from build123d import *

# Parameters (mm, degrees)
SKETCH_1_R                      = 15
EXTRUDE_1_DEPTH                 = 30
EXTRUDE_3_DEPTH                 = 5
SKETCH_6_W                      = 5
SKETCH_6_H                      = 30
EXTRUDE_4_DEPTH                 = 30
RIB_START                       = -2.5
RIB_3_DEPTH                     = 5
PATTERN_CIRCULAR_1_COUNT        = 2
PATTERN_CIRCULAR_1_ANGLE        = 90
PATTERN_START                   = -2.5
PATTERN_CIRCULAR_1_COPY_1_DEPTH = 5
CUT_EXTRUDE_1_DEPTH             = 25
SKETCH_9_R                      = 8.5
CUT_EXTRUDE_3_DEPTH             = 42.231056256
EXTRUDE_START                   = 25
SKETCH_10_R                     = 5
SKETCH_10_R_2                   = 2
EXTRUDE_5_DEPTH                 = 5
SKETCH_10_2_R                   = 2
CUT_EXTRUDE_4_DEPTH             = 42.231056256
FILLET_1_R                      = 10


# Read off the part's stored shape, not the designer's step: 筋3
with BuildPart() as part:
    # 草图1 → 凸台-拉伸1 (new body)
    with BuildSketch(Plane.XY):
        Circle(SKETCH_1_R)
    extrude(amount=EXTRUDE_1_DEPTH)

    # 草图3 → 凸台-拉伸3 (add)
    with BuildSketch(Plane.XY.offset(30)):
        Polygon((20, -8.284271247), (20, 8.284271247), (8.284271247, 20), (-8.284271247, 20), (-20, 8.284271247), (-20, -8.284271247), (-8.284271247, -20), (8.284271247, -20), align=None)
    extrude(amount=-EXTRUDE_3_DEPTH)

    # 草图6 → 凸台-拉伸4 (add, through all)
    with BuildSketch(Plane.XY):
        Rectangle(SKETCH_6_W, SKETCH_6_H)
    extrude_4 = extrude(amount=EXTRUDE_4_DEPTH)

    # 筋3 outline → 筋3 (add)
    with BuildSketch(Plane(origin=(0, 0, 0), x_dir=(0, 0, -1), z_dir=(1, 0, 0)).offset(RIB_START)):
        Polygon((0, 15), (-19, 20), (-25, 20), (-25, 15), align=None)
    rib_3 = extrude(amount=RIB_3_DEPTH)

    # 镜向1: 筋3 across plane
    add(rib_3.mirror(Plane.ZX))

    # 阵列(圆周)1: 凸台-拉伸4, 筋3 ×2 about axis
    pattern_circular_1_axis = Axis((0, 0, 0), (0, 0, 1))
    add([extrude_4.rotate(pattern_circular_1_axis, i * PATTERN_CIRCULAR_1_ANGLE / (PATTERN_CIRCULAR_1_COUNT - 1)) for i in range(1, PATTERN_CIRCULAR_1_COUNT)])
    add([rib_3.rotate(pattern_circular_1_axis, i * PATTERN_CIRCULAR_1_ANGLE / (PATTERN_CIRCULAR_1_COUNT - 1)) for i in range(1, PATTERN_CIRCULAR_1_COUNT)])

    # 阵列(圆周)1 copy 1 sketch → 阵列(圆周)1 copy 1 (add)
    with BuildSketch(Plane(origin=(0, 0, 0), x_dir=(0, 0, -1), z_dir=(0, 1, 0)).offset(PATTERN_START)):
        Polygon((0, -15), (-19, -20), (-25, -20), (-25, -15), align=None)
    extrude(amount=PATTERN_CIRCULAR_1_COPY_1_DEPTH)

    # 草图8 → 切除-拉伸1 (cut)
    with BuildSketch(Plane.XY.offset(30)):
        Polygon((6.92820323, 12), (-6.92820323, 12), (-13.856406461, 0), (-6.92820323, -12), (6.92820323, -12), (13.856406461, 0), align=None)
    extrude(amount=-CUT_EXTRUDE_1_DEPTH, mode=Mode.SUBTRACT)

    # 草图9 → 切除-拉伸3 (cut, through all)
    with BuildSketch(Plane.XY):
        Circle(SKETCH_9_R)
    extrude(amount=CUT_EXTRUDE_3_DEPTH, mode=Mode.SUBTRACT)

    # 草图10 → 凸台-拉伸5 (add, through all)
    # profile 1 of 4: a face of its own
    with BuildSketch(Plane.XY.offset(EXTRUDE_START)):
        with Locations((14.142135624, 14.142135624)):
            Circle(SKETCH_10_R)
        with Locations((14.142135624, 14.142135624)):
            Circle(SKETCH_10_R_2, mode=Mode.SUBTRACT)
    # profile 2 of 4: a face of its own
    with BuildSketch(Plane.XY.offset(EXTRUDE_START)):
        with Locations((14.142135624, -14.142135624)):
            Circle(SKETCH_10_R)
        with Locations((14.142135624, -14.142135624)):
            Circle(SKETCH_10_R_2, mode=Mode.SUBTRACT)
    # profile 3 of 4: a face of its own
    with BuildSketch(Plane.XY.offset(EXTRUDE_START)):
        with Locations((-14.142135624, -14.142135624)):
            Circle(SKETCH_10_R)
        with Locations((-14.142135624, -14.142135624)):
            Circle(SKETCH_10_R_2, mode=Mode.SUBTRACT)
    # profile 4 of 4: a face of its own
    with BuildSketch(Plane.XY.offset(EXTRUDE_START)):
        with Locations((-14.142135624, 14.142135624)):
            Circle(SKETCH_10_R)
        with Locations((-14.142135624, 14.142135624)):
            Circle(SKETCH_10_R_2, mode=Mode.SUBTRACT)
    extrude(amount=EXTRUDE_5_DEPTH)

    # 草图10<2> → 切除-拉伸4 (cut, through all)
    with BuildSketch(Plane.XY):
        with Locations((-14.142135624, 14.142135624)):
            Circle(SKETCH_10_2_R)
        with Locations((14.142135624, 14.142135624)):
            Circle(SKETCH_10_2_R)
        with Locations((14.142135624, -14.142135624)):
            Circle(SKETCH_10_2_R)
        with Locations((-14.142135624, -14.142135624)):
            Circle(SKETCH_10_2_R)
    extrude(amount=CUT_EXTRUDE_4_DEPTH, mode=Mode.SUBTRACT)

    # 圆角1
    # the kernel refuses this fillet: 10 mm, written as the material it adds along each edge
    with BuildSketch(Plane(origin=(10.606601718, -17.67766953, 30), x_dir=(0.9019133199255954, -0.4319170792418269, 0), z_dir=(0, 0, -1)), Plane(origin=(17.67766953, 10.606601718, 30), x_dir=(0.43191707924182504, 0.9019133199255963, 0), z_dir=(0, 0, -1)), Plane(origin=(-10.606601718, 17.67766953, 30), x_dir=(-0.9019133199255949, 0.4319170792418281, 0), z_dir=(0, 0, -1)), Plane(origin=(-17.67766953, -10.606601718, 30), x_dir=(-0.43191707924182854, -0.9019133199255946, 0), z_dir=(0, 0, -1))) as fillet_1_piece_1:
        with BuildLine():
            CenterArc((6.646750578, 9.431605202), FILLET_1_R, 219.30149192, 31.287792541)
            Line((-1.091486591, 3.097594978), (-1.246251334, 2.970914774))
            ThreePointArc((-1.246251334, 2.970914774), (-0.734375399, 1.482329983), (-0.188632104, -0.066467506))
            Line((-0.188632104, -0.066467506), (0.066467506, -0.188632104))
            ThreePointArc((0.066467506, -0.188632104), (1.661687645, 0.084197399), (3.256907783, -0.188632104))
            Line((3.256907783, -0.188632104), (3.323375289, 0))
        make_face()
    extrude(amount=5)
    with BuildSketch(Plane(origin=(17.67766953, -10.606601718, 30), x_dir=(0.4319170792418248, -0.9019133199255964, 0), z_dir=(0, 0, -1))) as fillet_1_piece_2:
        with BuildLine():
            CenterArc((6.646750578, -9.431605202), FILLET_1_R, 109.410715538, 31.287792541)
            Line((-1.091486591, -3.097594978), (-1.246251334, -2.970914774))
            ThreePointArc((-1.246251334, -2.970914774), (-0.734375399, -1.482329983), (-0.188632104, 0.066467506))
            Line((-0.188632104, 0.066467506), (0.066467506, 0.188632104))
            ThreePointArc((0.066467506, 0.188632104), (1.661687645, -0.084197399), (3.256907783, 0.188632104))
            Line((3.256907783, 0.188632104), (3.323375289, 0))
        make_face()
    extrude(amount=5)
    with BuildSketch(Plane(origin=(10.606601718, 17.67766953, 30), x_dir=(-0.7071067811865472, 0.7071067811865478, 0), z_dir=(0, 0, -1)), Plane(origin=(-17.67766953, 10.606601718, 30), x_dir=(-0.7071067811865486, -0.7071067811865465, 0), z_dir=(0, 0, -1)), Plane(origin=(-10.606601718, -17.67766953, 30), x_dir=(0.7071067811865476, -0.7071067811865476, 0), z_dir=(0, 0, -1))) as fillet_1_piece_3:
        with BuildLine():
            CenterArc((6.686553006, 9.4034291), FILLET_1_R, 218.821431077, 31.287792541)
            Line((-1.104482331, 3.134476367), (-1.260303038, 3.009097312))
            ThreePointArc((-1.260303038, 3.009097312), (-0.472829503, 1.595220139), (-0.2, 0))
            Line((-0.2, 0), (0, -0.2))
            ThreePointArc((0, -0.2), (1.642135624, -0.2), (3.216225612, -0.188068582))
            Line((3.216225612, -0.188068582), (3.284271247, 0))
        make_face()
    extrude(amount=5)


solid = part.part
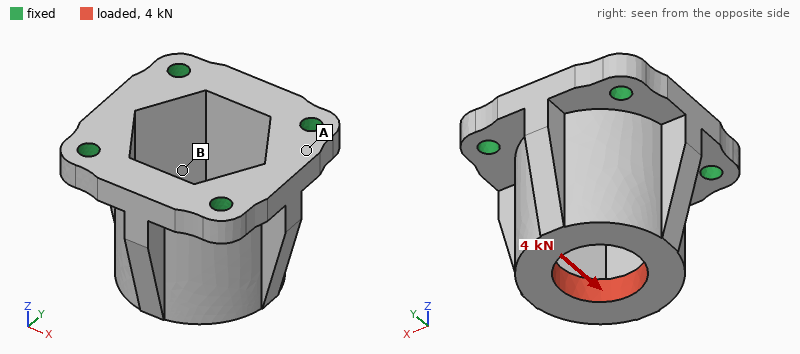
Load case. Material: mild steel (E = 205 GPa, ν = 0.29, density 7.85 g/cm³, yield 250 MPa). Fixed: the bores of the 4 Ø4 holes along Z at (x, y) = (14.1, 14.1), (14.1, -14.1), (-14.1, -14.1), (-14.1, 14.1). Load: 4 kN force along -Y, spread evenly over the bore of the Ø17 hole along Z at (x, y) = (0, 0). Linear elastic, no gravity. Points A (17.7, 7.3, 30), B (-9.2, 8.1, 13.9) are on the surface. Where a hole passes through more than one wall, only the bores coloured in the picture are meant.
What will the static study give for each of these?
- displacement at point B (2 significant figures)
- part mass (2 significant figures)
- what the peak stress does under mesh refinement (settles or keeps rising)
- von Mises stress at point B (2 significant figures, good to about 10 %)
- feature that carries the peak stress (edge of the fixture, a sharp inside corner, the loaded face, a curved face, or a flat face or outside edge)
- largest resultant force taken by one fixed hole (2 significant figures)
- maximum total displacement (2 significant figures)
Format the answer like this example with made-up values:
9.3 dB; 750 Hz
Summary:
12 µm; 100 g; keeps rising; 44 MPa; edge of the fixture; 2.2 kN; 27 µm
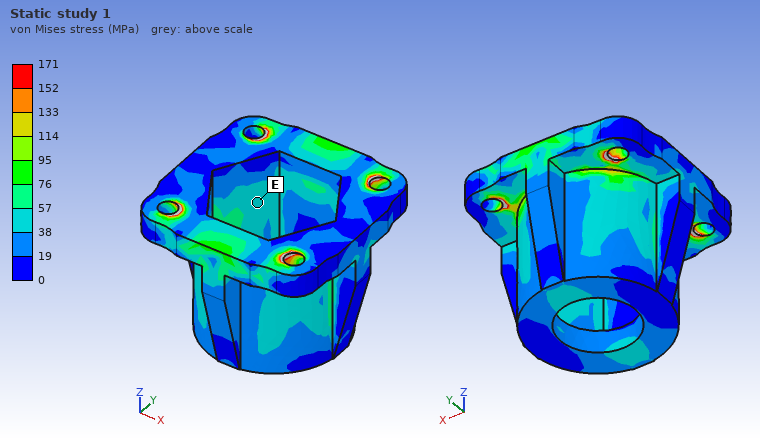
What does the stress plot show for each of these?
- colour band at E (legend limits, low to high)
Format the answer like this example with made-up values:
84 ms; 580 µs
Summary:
38 to 57 MPa
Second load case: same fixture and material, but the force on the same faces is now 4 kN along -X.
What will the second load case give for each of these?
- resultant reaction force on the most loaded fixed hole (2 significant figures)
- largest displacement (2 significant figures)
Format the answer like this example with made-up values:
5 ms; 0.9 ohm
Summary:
2.1 kN; 28 µm
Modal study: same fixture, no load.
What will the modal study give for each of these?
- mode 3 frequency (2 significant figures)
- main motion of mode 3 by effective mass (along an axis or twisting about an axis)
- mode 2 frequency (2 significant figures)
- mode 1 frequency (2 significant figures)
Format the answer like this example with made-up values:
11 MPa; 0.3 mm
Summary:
19 kHz; along Z; 11 kHz; 11 kHz
